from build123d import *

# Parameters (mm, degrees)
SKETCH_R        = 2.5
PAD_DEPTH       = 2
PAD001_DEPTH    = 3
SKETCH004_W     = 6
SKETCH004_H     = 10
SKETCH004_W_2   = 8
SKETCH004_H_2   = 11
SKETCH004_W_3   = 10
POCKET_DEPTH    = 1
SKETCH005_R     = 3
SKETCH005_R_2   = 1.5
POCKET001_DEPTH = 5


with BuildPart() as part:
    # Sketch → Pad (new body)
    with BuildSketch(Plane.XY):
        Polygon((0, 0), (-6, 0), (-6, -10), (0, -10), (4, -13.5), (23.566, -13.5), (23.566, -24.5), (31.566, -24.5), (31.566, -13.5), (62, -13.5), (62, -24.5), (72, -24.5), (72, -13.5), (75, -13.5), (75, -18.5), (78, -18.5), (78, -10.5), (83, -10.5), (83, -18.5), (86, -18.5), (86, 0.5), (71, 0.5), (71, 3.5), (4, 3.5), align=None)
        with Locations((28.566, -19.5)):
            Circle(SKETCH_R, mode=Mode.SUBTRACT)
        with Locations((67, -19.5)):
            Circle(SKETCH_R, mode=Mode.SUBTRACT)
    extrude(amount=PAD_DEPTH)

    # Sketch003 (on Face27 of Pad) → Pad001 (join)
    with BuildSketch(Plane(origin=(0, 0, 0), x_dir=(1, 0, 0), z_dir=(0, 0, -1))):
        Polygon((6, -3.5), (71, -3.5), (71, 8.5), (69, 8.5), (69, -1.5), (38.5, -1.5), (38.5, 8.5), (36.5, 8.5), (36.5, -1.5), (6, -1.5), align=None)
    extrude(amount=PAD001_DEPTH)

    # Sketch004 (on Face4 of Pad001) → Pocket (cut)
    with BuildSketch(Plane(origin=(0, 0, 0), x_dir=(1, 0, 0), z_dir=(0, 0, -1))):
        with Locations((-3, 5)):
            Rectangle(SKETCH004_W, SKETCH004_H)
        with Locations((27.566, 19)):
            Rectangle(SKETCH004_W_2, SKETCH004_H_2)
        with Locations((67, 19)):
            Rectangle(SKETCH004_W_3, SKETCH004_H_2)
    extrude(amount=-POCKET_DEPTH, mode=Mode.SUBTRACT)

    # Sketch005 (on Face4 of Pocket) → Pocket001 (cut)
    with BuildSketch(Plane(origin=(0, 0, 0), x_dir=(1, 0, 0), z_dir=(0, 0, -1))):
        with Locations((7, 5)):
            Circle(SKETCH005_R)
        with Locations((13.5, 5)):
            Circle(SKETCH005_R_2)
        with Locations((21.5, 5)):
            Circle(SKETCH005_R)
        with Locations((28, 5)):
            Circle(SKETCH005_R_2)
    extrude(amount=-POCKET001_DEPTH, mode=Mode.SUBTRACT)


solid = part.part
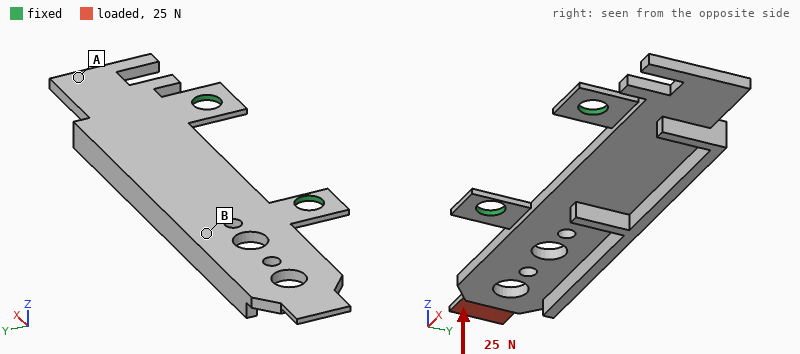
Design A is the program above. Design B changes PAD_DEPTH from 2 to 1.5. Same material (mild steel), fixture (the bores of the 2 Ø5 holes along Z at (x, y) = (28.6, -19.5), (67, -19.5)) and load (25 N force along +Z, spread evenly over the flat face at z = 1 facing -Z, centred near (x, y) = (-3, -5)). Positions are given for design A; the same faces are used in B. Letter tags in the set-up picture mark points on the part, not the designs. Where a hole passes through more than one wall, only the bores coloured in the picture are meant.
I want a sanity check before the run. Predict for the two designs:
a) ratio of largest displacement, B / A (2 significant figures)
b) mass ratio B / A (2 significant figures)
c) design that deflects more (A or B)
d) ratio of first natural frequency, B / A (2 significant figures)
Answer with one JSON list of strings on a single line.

["3.5", "0.77", "B", "0.42"]
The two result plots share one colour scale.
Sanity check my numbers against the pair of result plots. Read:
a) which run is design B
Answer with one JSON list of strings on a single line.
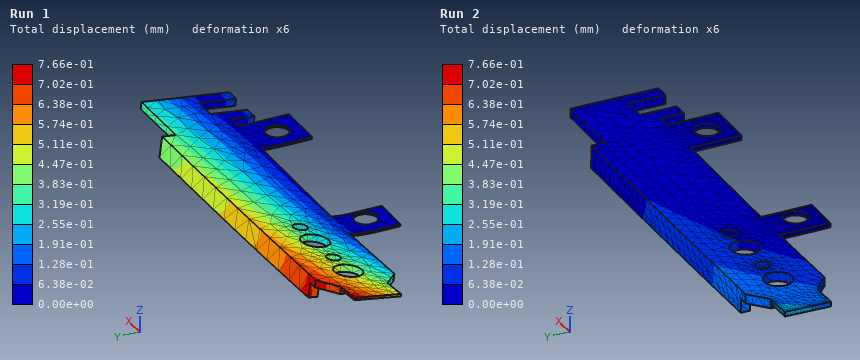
["Run 1"]
